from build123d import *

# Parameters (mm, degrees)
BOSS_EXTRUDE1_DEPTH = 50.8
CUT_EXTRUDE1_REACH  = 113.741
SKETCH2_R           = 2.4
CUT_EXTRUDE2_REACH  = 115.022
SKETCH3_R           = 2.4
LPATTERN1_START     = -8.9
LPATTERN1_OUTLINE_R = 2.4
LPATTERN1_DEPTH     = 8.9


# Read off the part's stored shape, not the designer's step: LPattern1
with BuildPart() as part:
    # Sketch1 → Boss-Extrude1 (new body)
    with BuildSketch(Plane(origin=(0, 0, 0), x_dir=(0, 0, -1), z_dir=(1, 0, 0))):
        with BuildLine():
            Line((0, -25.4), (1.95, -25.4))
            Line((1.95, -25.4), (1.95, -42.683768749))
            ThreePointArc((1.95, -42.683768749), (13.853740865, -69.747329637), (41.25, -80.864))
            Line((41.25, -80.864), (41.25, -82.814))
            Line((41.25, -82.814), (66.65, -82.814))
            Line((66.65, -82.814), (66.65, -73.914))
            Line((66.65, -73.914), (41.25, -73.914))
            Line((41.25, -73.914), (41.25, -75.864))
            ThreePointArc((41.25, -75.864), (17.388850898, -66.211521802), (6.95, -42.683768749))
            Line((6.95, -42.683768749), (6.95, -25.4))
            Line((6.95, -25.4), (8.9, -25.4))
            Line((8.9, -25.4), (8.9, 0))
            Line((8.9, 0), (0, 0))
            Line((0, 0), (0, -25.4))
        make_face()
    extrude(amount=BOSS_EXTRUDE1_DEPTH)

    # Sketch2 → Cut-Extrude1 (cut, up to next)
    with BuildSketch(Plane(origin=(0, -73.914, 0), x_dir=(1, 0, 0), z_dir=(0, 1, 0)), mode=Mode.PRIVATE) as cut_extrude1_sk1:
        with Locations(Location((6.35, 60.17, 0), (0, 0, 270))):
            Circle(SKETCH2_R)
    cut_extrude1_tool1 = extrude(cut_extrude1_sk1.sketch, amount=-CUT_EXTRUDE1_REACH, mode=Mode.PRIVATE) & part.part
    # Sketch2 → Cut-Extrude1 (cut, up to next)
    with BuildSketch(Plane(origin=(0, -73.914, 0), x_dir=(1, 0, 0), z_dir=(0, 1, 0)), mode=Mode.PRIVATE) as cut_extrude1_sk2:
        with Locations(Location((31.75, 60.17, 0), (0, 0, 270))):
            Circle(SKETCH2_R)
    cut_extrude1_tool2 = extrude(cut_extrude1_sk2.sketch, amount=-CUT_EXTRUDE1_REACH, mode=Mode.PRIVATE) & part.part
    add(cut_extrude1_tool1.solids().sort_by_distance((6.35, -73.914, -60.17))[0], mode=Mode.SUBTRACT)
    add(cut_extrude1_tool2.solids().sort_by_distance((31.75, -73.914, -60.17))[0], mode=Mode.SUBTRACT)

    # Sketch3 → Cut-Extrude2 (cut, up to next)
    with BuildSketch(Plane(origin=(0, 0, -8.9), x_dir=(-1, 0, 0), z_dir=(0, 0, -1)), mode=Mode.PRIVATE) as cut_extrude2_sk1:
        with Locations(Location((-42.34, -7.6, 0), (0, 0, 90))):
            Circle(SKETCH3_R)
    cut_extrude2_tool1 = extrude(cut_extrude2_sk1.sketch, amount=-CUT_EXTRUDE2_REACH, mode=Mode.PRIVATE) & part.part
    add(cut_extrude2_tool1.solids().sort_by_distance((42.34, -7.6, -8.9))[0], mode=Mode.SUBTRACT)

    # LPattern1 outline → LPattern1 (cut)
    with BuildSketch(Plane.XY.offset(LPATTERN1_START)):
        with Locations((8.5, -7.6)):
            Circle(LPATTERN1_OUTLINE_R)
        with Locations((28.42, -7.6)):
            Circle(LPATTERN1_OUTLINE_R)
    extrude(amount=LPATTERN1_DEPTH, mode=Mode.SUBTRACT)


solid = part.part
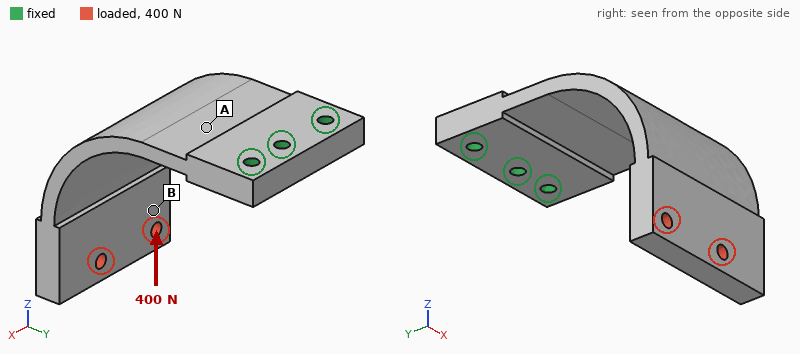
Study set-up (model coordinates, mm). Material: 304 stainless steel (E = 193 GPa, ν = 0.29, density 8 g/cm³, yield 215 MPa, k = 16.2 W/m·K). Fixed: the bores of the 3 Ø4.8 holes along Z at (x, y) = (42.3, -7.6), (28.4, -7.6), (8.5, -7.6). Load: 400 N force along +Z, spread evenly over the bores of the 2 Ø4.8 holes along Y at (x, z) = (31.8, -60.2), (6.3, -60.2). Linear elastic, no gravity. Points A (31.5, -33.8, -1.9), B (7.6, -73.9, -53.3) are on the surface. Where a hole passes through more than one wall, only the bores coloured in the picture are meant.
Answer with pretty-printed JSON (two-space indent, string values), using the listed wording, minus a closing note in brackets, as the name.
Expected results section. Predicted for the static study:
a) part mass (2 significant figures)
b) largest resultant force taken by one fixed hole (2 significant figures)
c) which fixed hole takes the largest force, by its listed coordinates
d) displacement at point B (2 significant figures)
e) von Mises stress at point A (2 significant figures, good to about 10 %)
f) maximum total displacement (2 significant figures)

{
  "part mass": "330 g",
  "largest resultant force taken by one fixed hole": "310 N",
  "which fixed hole takes the largest force, by its listed coordinates": "(28.4, -7.6)",
  "displacement at point B": "0.38 mm",
  "von Mises stress at point A": "73 MPa",
  "maximum total displacement": "0.49 mm"
}
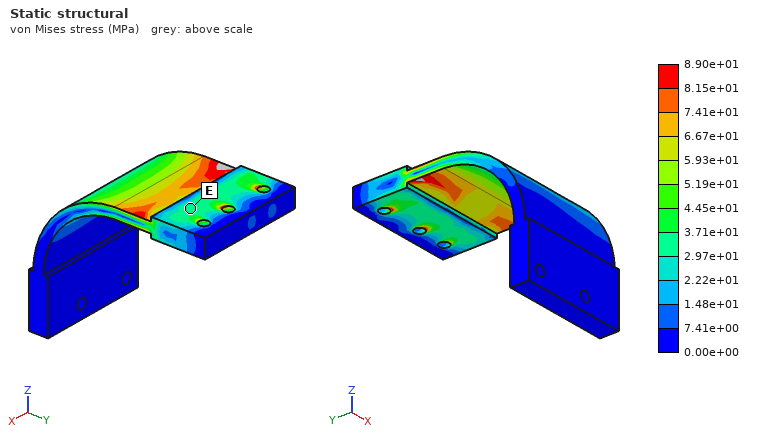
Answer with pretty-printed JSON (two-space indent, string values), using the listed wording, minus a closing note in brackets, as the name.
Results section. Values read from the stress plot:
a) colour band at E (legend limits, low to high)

{
  "colour band at E": "2.97e+01 to 3.71e+01 MPa"
}
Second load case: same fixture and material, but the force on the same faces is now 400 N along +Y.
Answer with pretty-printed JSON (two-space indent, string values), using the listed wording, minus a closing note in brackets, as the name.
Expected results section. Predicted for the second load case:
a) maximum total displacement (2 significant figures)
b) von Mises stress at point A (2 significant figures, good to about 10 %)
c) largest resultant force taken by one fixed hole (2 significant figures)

{
  "maximum total displacement": "0.86 mm",
  "von Mises stress at point A": "90 MPa",
  "largest resultant force taken by one fixed hole": "250 N"
}
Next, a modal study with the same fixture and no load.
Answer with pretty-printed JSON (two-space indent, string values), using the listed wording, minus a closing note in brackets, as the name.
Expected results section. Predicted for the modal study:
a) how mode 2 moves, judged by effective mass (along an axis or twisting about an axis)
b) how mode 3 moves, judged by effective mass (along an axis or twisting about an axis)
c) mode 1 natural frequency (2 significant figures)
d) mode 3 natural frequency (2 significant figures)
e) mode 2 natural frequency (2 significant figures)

{
  "how mode 2 moves, judged by effective mass": "along X",
  "how mode 3 moves, judged by effective mass": "along Z",
  "mode 1 natural frequency": "350 Hz",
  "mode 3 natural frequency": "1300 Hz",
  "mode 2 natural frequency": "690 Hz"
}
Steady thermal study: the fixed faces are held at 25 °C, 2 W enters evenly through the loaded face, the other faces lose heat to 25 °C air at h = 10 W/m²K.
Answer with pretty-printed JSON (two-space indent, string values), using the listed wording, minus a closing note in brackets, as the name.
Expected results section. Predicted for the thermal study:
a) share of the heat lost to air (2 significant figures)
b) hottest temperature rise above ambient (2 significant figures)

{
  "share of the heat lost to air": "70 %",
  "hottest temperature rise above ambient": "24 K"
}
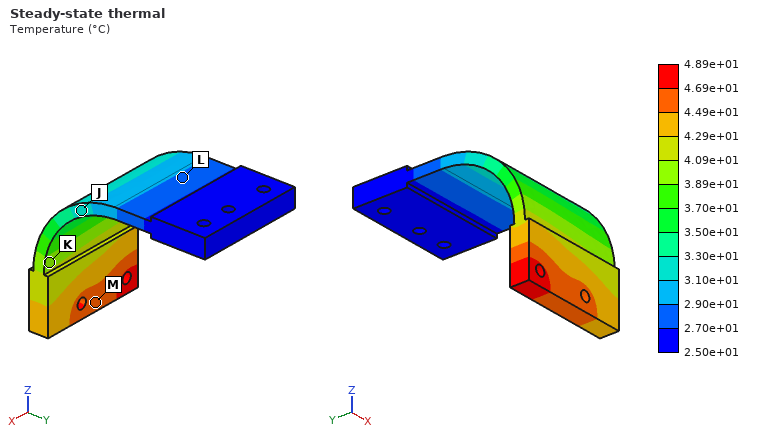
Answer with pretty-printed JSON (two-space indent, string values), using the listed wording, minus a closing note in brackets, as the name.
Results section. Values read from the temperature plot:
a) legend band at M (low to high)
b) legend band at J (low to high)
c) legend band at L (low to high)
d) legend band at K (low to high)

{
  "legend band at M": "4.49e+01 to 4.69e+01 °C",
  "legend band at J": "3.10e+01 to 3.30e+01 °C",
  "legend band at L": "2.70e+01 to 2.90e+01 °C",
  "legend band at K": "3.89e+01 to 4.09e+01 °C"
}
